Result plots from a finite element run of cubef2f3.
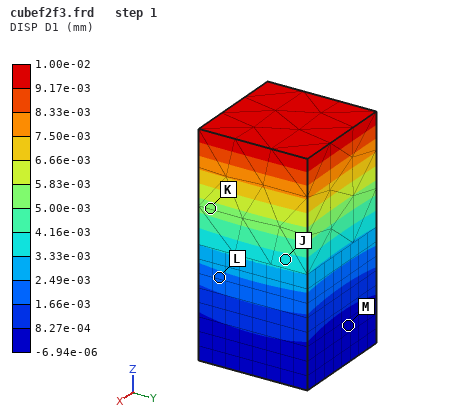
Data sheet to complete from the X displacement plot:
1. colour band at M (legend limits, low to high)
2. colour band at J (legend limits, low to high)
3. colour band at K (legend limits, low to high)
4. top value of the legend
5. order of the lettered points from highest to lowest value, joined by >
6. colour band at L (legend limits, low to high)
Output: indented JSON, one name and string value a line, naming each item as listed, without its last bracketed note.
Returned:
{
  "colour band at M": "-6.94e-06 to 8.27e-04 mm",
  "colour band at J": "3.33e-03 to 4.16e-03 mm",
  "colour band at K": "5.00e-03 to 5.83e-03 mm",
  "top value of the legend": "1.00e-02 mm",
  "order of the lettered points from highest to lowest value, joined by >": "K > J > L > M",
  "colour band at L": "1.66e-03 to 2.49e-03 mm"
}
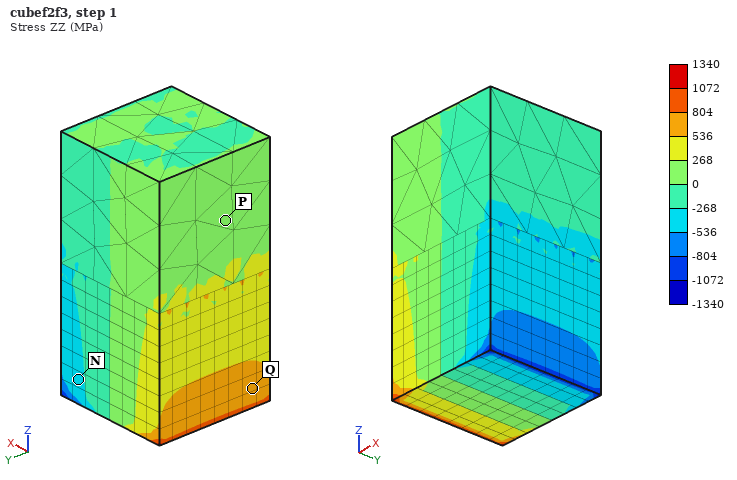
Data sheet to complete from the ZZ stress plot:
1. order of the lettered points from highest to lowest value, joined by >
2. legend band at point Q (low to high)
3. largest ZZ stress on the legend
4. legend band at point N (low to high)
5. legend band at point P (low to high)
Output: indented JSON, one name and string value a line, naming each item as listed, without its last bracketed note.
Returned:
{
  "order of the lettered points from highest to lowest value, joined by >": "Q > P > N",
  "legend band at point Q": "536 to 804 MPa",
  "largest ZZ stress on the legend": "1340 MPa",
  "legend band at point N": "-536 to -268 MPa",
  "legend band at point P": "0 to 268 MPa"
}
